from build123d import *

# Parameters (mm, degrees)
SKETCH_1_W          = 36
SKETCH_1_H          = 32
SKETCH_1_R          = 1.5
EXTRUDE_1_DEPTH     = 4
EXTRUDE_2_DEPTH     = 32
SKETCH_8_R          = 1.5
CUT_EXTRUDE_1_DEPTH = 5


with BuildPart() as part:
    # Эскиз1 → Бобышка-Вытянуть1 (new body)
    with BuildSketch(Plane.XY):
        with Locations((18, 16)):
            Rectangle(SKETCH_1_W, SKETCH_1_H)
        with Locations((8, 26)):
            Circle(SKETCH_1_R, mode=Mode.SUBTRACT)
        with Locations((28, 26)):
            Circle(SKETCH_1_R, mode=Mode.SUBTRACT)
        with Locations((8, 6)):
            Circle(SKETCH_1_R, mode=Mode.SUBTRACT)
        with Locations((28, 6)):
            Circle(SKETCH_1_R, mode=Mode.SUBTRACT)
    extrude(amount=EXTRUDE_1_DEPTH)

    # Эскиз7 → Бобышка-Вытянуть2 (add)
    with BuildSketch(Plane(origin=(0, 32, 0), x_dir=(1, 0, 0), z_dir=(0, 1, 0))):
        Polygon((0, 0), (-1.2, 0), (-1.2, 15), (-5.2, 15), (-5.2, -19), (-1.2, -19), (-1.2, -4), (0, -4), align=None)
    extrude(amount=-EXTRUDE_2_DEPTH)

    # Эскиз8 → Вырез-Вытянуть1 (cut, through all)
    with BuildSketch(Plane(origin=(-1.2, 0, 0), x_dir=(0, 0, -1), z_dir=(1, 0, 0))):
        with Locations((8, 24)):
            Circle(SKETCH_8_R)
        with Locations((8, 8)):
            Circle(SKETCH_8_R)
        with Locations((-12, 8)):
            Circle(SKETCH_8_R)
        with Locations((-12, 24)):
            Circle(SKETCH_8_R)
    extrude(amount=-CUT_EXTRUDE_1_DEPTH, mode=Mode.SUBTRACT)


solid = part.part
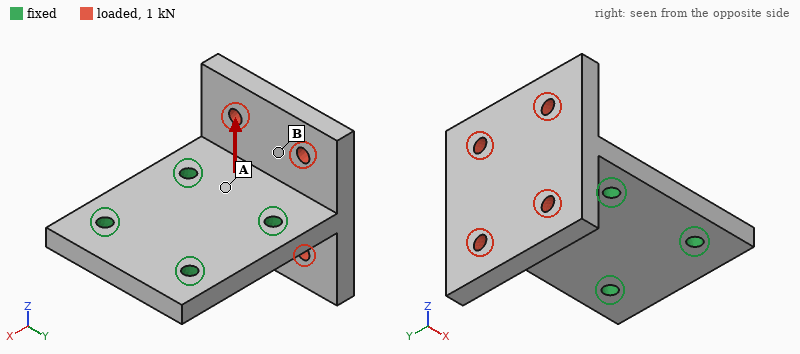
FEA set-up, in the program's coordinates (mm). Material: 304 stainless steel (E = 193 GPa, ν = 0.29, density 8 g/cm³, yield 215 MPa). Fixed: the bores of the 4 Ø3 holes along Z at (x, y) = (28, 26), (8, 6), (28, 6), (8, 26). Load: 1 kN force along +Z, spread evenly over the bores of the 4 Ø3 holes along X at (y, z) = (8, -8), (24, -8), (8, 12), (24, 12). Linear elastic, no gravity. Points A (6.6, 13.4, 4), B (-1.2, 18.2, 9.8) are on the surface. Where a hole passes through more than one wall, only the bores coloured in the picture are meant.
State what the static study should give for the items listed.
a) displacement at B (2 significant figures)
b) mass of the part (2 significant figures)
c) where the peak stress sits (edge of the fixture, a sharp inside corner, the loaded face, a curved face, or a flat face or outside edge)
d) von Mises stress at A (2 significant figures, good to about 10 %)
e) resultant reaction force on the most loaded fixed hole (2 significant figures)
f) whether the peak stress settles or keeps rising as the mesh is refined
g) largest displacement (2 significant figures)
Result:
20 µm
71 g
edge of the fixture
57 MPa
570 N
keeps rising
40 µm
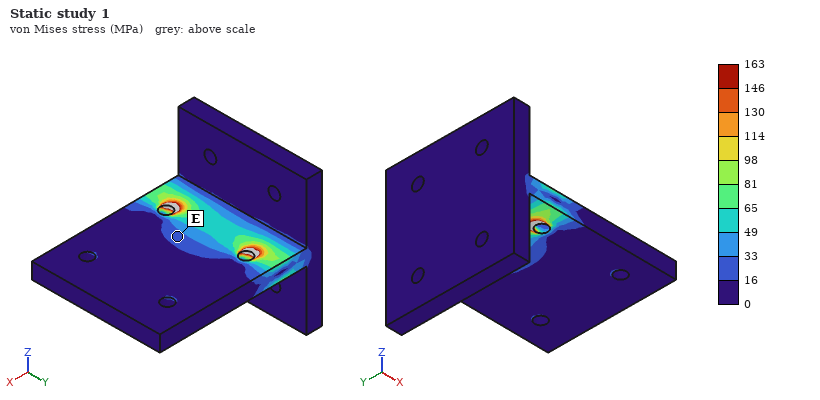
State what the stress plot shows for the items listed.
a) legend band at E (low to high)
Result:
16 to 33 MPa
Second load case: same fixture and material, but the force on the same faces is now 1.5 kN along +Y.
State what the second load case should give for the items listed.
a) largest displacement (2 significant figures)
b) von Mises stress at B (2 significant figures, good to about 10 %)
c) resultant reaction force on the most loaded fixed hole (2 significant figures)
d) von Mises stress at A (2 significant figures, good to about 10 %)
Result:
3.9 µm
10 MPa
990 N
17 MPa
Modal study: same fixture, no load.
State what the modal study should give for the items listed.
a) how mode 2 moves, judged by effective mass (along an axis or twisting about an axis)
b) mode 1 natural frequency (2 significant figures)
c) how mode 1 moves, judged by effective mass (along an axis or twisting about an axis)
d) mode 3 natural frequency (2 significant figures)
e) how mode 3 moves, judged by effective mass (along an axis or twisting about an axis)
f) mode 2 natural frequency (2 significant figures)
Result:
twisting about X
4000 Hz
along Z
12 kHz
along X
7700 Hz
